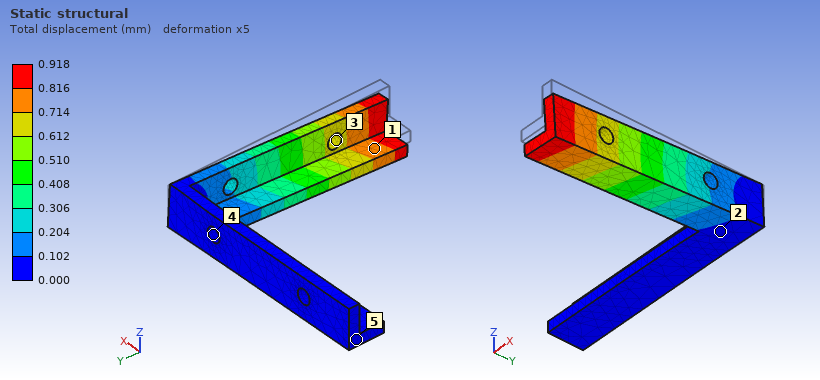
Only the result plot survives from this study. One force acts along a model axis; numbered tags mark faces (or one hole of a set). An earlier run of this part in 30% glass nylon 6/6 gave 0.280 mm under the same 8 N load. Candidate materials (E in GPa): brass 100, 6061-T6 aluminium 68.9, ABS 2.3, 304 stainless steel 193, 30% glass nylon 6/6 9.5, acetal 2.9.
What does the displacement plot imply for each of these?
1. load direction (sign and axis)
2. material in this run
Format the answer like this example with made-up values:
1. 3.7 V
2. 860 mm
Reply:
1. -Z
2. acetal
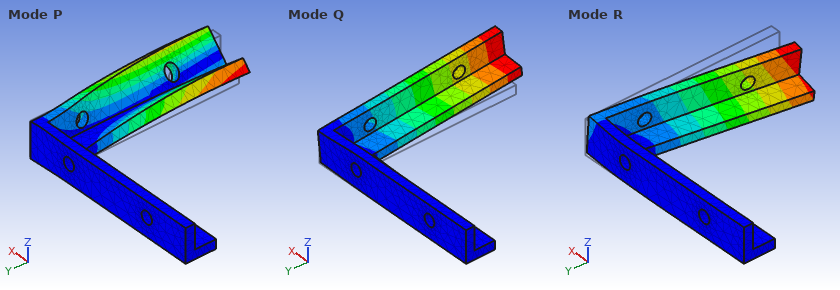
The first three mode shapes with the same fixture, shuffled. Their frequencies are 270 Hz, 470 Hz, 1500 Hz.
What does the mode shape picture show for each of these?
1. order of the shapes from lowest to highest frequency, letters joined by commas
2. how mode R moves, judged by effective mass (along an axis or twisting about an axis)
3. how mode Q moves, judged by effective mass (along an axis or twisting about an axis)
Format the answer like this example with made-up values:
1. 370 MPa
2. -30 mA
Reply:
1. Q, R, P
2. along X
3. along Z
